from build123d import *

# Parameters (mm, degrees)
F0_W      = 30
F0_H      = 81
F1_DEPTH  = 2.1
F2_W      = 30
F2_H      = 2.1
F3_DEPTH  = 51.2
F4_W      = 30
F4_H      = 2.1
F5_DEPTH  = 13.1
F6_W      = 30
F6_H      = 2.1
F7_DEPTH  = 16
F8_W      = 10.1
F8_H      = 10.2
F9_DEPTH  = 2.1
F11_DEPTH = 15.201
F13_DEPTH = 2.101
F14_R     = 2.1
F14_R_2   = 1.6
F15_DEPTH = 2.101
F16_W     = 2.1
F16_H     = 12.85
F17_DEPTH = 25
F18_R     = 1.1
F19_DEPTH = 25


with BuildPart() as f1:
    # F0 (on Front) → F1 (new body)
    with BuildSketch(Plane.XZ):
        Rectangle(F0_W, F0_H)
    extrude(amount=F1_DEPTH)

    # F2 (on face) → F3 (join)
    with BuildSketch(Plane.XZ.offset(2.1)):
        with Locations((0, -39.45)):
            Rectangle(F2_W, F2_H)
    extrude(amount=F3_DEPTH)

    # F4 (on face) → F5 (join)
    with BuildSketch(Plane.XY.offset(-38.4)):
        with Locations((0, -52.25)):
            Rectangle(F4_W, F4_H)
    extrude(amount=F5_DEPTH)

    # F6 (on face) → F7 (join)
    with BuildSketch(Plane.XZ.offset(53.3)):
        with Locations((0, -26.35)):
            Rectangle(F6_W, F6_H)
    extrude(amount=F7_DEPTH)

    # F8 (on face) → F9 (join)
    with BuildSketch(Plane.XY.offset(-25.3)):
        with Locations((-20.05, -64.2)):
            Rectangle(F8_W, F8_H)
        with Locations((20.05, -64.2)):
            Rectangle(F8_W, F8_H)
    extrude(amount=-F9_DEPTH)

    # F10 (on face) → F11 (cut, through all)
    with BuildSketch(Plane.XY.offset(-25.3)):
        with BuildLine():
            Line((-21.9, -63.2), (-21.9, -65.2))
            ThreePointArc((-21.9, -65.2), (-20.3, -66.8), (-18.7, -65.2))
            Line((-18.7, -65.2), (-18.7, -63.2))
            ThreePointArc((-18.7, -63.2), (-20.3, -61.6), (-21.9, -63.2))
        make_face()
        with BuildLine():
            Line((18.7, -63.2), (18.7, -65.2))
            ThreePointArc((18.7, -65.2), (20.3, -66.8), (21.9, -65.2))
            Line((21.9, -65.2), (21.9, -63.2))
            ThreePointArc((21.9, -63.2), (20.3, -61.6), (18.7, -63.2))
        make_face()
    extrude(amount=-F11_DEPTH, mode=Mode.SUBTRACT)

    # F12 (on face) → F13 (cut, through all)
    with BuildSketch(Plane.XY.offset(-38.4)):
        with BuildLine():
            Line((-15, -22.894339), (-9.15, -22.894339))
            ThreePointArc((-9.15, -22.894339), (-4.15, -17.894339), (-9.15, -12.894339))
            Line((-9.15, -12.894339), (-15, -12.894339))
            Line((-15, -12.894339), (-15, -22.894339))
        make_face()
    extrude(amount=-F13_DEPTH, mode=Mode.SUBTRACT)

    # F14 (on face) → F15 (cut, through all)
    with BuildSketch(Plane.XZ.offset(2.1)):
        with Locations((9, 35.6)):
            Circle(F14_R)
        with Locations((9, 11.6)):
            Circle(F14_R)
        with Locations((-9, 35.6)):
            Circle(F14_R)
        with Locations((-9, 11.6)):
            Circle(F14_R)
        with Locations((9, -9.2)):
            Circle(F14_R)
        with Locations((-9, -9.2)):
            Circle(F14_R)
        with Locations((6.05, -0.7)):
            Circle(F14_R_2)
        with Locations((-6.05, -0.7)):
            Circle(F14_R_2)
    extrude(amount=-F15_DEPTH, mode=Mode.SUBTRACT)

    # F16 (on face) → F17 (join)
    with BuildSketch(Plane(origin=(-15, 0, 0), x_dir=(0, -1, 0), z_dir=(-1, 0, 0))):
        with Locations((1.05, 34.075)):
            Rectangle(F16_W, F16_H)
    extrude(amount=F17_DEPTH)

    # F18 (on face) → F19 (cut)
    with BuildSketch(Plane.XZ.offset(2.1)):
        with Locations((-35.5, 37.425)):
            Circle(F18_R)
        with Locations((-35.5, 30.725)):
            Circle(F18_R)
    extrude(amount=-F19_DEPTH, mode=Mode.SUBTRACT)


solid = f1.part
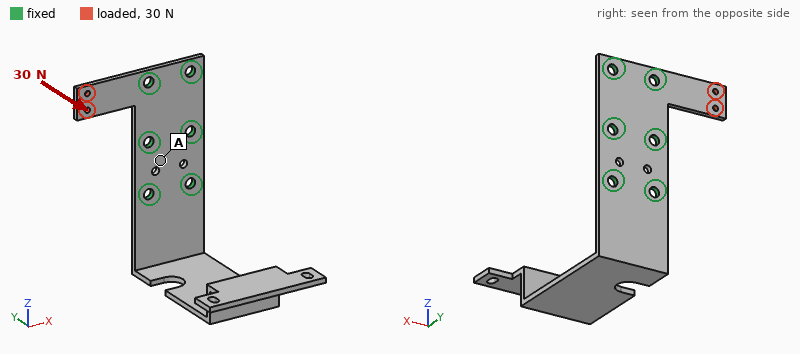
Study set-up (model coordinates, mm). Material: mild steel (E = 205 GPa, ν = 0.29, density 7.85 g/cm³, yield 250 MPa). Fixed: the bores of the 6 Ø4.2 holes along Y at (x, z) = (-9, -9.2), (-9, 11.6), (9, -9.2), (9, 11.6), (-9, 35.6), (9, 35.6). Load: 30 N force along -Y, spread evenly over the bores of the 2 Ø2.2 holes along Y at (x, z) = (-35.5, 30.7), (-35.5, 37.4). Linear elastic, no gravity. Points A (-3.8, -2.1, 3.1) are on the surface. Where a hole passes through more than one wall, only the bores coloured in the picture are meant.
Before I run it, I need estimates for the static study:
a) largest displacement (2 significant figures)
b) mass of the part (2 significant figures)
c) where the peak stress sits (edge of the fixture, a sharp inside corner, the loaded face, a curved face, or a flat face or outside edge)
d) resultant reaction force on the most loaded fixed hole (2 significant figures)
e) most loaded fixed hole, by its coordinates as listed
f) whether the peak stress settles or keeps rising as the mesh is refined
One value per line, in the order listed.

95 µm
85 g
edge of the fixture
36 N
(-9, 35.6)
keeps rising
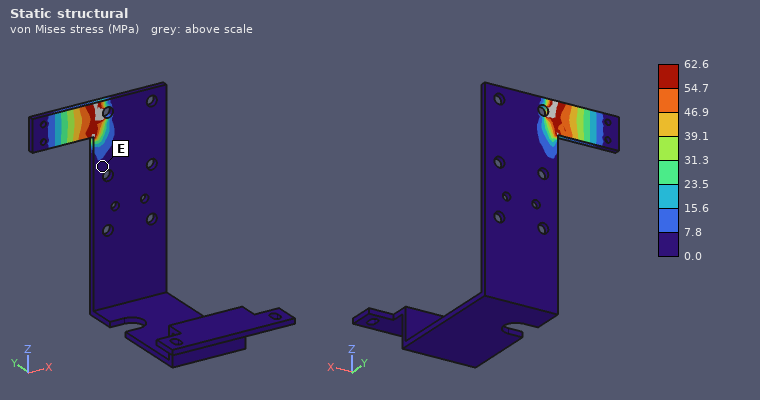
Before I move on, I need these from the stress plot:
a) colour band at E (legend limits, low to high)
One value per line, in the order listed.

0.0 to 7.8 MPa
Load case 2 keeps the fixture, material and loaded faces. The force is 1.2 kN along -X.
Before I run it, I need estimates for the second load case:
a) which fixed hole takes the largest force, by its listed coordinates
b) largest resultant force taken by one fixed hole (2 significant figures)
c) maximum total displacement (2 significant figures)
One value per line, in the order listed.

(-9, 35.6)
1.0 kN
6.3 µm
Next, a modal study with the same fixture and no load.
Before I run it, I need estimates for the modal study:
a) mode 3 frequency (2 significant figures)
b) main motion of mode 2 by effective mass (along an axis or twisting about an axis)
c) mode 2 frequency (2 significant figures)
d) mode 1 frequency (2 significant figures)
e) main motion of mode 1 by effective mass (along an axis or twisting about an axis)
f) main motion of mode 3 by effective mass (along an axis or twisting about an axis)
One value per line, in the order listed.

650 Hz
along X
320 Hz
170 Hz
along Z
along Y
